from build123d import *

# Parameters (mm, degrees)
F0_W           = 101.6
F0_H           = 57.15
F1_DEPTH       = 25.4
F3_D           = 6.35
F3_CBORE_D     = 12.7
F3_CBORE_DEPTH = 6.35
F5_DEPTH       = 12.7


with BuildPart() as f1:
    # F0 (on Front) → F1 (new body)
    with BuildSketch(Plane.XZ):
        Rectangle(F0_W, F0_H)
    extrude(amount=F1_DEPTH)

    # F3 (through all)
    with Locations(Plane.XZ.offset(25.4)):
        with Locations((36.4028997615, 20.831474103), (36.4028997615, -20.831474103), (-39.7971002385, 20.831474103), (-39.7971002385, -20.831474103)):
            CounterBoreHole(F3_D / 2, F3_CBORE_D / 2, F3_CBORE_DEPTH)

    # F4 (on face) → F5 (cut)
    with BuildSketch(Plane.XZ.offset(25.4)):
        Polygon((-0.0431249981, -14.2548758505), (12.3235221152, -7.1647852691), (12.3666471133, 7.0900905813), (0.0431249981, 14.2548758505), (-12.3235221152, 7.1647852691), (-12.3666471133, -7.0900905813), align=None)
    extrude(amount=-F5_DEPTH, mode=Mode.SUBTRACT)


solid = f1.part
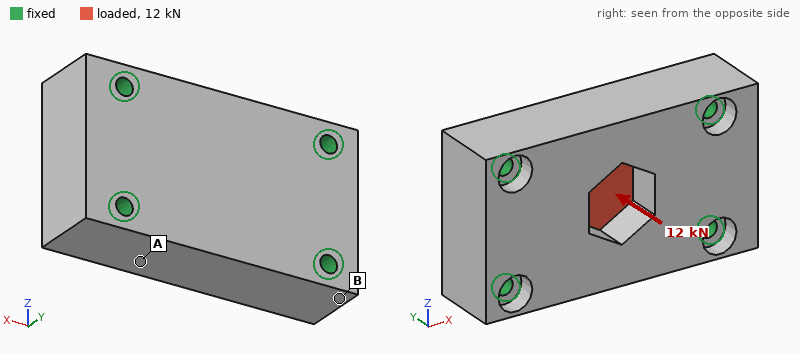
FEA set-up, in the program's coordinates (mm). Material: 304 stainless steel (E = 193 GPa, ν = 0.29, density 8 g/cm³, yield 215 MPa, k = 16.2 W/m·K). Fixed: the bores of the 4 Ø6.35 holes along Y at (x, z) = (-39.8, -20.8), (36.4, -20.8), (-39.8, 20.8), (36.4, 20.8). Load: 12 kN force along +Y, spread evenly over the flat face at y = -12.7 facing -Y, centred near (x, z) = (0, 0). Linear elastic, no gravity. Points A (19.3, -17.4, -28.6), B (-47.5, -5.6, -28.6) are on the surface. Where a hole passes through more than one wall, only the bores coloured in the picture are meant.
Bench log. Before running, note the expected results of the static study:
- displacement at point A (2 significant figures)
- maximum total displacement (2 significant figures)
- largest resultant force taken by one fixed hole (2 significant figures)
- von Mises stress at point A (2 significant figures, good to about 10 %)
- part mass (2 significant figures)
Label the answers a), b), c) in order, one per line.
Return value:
a) 2.8 µm
b) 8.8 µm
c) 3.2 kN
d) 9.7 MPa
e) 1.1 kg
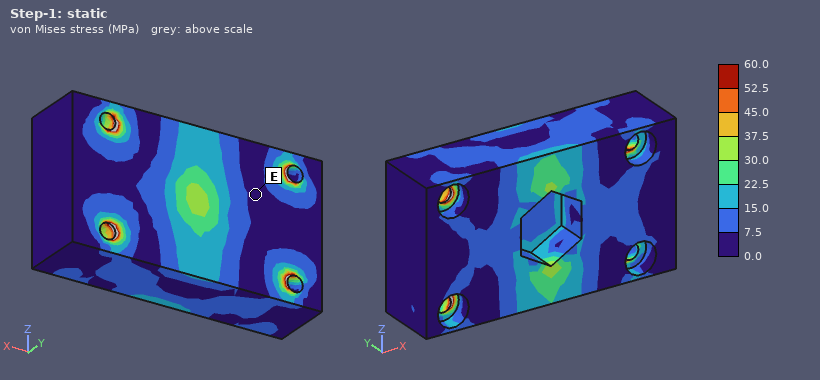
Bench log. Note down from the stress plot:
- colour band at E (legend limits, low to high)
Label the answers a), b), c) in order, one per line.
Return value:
a) 0.0 to 7.5 MPa
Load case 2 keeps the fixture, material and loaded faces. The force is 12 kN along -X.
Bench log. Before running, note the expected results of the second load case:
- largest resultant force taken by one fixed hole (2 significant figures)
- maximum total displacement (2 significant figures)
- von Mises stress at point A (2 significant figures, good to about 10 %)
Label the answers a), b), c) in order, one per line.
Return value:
a) 3.2 kN
b) 3.4 µm
c) 3.3 MPa
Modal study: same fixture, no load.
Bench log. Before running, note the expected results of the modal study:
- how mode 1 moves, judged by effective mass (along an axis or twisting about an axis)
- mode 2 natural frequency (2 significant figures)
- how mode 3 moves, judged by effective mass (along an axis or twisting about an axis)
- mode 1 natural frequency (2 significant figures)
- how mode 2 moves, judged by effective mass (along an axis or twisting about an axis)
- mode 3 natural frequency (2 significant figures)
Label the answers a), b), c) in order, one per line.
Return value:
a) along Y
b) 16 kHz
c) along Z
d) 11 kHz
e) twisting about X
f) 17 kHz
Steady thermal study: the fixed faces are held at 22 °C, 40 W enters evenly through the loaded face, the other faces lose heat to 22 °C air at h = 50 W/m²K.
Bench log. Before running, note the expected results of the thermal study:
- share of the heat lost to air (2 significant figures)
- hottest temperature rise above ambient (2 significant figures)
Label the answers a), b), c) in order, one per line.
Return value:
a) 27 %
b) 63 K
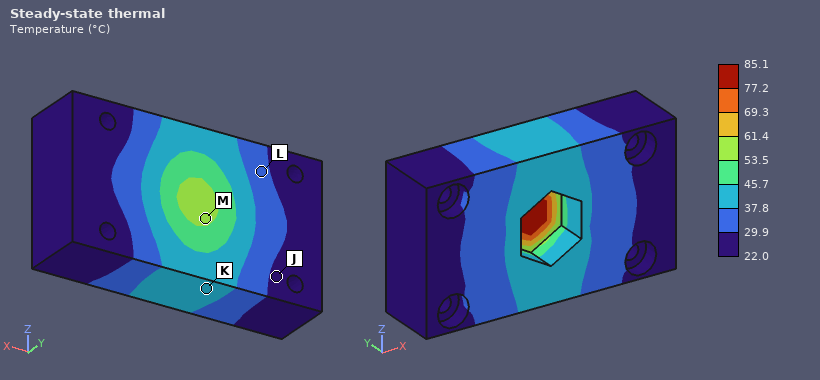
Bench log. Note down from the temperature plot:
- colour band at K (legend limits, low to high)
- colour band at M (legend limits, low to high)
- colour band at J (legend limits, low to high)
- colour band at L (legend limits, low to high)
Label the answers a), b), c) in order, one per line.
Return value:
a) 37.8 to 45.7 °C
b) 53.5 to 61.4 °C
c) 22.0 to 29.9 °C
d) 29.9 to 37.8 °C
